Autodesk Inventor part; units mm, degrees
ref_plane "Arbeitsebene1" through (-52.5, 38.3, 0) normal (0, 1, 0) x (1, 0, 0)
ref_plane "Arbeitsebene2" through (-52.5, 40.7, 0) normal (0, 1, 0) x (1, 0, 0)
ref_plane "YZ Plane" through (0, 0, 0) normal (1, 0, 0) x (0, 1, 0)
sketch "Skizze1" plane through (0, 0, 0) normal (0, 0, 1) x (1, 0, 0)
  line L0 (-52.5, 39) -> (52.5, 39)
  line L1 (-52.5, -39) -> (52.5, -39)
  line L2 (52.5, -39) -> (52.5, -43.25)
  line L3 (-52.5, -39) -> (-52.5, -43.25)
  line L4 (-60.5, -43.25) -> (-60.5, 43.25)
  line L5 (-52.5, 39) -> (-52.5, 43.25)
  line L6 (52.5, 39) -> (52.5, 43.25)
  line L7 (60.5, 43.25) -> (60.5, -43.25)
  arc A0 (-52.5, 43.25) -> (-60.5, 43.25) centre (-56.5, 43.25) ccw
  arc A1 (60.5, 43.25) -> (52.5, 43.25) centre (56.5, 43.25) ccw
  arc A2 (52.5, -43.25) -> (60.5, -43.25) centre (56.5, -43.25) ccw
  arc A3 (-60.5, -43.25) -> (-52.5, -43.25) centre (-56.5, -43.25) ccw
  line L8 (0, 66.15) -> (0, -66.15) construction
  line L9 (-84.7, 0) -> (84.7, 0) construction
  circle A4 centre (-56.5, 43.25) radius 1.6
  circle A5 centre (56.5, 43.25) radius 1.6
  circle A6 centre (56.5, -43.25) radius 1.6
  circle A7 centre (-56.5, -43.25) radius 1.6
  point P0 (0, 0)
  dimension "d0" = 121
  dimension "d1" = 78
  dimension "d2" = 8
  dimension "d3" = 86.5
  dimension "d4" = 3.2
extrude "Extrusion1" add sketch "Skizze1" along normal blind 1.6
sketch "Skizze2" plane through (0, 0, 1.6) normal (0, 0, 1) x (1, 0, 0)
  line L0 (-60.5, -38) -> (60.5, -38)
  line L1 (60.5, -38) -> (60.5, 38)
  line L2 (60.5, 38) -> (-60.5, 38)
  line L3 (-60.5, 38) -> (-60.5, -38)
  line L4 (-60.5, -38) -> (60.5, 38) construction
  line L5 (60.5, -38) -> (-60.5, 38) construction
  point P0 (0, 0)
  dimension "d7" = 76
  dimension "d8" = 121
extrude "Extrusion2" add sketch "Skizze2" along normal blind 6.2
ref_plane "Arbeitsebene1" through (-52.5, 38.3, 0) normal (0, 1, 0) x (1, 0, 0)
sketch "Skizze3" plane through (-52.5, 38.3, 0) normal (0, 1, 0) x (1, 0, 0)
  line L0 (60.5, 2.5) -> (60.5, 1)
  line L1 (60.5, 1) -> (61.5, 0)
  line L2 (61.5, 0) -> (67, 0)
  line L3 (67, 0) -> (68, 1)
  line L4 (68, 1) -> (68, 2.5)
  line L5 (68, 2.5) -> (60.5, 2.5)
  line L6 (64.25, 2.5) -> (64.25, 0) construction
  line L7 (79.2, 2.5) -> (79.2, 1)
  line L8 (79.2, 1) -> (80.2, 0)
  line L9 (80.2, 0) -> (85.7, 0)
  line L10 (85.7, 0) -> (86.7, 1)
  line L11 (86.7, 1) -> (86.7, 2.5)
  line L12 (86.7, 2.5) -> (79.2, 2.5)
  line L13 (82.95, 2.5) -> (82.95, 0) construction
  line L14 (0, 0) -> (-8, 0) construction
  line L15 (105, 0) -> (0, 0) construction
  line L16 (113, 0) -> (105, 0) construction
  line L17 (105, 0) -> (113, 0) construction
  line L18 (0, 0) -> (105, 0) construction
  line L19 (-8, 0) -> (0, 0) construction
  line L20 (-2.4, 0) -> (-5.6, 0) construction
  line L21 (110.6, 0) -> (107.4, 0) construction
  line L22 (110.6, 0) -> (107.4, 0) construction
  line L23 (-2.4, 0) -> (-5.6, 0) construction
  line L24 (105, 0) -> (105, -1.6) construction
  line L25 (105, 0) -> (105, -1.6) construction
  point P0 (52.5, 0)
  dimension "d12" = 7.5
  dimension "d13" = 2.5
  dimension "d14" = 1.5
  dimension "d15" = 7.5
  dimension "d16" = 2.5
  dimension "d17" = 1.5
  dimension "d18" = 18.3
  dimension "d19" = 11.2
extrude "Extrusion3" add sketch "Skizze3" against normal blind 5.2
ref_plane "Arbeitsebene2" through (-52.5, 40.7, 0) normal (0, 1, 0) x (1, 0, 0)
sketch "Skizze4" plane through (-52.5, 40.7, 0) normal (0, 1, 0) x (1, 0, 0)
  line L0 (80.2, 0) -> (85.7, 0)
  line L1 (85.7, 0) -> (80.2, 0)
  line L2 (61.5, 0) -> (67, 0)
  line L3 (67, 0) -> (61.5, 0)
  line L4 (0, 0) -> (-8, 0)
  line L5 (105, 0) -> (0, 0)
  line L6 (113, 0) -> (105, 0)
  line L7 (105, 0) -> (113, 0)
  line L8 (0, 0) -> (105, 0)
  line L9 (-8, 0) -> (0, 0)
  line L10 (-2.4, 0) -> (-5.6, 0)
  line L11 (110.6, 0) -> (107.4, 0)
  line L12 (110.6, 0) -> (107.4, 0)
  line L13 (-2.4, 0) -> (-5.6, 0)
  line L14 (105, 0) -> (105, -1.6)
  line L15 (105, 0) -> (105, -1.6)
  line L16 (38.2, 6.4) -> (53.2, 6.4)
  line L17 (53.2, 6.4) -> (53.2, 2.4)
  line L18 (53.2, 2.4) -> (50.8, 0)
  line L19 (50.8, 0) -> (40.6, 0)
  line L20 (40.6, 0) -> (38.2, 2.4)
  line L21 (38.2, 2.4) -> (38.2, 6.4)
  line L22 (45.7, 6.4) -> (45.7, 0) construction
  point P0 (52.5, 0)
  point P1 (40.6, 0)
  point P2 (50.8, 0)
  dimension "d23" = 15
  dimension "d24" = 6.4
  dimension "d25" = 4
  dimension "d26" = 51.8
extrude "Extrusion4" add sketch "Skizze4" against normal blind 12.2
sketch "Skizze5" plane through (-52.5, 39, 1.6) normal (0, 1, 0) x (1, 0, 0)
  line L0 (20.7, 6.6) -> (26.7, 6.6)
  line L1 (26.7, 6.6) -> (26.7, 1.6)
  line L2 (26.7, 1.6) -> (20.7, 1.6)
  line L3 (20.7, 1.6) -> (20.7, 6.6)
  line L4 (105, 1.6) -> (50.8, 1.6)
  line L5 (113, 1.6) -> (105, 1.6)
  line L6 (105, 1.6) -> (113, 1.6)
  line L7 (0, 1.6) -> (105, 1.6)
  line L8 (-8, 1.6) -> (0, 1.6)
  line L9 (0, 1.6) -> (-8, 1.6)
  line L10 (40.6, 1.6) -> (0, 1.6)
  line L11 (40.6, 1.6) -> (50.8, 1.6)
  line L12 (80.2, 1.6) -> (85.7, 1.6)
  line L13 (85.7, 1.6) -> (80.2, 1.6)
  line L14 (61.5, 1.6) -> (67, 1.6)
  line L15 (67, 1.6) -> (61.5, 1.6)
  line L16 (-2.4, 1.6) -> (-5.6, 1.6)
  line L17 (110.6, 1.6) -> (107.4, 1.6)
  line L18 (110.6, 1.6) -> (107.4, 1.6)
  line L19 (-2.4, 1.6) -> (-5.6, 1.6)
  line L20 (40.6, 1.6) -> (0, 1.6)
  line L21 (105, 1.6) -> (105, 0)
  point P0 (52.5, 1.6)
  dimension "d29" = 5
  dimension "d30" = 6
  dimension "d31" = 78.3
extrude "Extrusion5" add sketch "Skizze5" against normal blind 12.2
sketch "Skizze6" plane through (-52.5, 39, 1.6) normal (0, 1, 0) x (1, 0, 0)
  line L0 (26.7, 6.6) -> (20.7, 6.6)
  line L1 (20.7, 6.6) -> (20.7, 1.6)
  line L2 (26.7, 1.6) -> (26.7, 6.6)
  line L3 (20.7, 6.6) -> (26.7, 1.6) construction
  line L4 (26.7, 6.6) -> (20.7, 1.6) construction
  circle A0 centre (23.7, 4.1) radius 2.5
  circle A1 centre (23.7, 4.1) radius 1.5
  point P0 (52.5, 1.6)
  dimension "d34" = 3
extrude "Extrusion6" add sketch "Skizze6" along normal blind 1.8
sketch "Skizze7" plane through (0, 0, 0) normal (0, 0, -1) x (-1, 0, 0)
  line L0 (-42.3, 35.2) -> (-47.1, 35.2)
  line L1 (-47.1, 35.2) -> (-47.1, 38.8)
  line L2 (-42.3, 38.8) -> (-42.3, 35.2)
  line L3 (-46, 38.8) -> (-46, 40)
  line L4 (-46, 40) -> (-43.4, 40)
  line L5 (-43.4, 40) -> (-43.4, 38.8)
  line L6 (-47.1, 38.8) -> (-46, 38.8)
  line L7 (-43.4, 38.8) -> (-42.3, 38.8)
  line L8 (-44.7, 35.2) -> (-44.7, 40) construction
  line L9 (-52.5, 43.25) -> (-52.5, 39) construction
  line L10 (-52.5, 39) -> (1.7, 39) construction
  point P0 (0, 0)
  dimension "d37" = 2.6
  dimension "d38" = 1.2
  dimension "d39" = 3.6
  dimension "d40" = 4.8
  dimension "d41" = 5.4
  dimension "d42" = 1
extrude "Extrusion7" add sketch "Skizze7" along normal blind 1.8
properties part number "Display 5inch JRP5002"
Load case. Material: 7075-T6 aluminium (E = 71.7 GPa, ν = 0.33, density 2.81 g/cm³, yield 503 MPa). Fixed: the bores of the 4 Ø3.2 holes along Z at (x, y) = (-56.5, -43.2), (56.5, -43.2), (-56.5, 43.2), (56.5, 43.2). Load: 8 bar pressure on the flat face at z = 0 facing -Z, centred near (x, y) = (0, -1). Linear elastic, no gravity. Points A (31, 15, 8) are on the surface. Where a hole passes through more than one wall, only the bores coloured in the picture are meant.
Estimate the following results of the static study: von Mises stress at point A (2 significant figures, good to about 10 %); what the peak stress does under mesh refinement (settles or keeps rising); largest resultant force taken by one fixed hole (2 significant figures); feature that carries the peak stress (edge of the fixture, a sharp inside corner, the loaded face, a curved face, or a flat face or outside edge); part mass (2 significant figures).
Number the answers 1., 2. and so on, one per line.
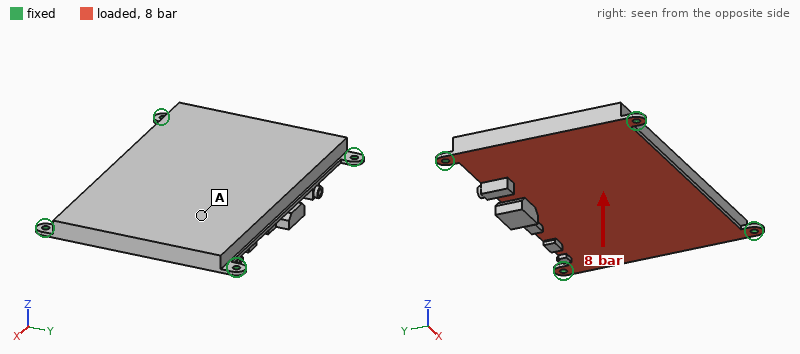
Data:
1. 69 MPa
2. keeps rising
3. 3.5 kN
4. edge of the fixture
5. 210 g
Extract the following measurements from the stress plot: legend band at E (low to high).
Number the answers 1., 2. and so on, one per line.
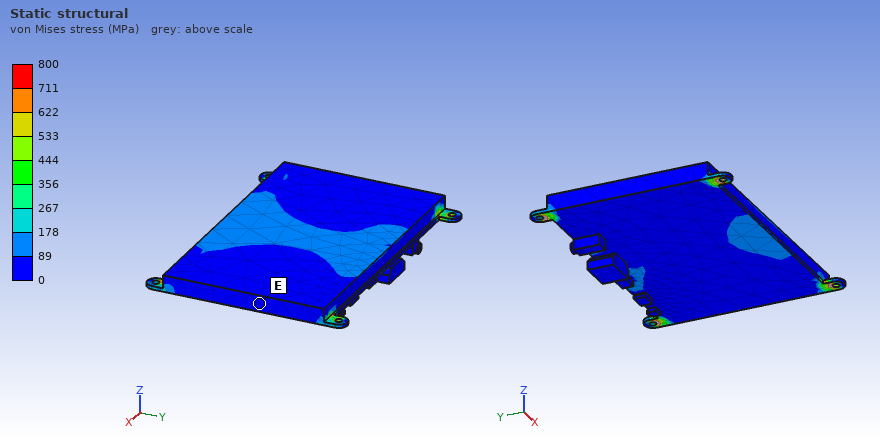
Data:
1. 0 to 89 MPa
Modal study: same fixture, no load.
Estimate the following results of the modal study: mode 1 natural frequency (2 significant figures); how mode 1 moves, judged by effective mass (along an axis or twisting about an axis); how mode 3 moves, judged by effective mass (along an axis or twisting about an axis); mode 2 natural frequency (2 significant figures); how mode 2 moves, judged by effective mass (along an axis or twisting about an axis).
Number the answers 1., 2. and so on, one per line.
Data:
1. 1300 Hz
2. along Z
3. twisting about Y
4. 2600 Hz
5. twisting about X
